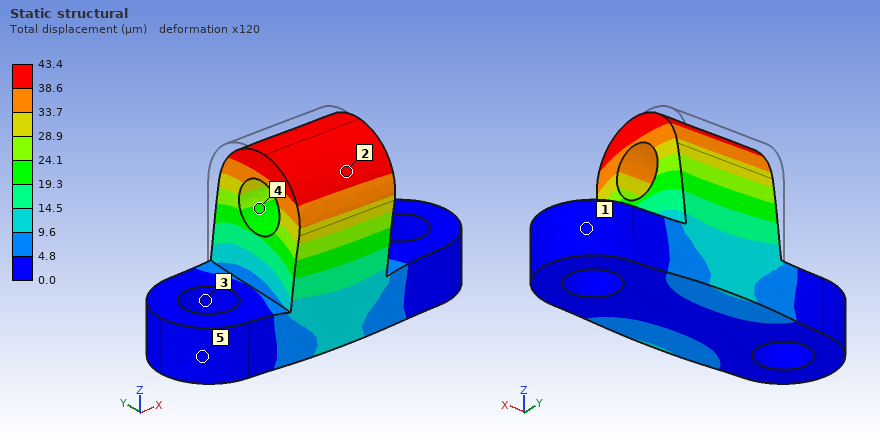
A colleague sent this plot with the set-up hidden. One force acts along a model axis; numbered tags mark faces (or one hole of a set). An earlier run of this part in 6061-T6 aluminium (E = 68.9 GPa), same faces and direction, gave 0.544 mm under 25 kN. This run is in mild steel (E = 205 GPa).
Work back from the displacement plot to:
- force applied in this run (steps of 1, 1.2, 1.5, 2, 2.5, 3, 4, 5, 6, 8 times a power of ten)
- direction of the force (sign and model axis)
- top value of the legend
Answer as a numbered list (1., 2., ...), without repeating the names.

1. 6 kN
2. -Y
3. 43.4 µm
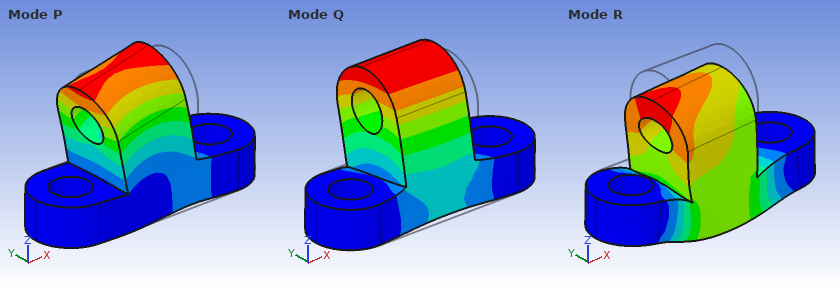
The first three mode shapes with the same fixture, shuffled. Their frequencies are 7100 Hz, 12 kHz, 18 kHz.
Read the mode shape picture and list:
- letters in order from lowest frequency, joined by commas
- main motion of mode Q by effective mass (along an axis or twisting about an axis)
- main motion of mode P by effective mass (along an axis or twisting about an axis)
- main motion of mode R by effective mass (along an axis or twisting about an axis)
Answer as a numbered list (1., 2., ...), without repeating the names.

1. Q, P, R
2. along Y
3. along X
4. along Z
